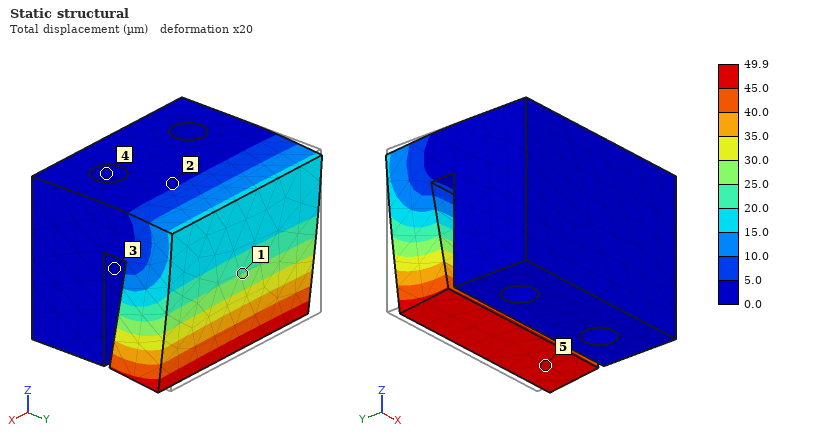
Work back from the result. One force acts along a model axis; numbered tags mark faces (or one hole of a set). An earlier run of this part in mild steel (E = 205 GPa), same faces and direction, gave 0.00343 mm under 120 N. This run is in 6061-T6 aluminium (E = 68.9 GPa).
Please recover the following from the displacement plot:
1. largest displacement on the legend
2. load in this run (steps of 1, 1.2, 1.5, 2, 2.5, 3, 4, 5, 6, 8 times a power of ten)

49.9 µm
600 N
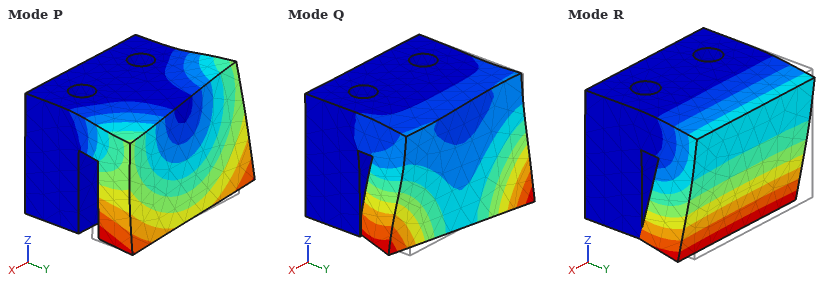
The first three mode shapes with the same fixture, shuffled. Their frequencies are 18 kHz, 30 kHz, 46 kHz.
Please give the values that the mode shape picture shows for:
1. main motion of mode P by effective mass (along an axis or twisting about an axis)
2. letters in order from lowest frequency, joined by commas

along X
R, P, Q
